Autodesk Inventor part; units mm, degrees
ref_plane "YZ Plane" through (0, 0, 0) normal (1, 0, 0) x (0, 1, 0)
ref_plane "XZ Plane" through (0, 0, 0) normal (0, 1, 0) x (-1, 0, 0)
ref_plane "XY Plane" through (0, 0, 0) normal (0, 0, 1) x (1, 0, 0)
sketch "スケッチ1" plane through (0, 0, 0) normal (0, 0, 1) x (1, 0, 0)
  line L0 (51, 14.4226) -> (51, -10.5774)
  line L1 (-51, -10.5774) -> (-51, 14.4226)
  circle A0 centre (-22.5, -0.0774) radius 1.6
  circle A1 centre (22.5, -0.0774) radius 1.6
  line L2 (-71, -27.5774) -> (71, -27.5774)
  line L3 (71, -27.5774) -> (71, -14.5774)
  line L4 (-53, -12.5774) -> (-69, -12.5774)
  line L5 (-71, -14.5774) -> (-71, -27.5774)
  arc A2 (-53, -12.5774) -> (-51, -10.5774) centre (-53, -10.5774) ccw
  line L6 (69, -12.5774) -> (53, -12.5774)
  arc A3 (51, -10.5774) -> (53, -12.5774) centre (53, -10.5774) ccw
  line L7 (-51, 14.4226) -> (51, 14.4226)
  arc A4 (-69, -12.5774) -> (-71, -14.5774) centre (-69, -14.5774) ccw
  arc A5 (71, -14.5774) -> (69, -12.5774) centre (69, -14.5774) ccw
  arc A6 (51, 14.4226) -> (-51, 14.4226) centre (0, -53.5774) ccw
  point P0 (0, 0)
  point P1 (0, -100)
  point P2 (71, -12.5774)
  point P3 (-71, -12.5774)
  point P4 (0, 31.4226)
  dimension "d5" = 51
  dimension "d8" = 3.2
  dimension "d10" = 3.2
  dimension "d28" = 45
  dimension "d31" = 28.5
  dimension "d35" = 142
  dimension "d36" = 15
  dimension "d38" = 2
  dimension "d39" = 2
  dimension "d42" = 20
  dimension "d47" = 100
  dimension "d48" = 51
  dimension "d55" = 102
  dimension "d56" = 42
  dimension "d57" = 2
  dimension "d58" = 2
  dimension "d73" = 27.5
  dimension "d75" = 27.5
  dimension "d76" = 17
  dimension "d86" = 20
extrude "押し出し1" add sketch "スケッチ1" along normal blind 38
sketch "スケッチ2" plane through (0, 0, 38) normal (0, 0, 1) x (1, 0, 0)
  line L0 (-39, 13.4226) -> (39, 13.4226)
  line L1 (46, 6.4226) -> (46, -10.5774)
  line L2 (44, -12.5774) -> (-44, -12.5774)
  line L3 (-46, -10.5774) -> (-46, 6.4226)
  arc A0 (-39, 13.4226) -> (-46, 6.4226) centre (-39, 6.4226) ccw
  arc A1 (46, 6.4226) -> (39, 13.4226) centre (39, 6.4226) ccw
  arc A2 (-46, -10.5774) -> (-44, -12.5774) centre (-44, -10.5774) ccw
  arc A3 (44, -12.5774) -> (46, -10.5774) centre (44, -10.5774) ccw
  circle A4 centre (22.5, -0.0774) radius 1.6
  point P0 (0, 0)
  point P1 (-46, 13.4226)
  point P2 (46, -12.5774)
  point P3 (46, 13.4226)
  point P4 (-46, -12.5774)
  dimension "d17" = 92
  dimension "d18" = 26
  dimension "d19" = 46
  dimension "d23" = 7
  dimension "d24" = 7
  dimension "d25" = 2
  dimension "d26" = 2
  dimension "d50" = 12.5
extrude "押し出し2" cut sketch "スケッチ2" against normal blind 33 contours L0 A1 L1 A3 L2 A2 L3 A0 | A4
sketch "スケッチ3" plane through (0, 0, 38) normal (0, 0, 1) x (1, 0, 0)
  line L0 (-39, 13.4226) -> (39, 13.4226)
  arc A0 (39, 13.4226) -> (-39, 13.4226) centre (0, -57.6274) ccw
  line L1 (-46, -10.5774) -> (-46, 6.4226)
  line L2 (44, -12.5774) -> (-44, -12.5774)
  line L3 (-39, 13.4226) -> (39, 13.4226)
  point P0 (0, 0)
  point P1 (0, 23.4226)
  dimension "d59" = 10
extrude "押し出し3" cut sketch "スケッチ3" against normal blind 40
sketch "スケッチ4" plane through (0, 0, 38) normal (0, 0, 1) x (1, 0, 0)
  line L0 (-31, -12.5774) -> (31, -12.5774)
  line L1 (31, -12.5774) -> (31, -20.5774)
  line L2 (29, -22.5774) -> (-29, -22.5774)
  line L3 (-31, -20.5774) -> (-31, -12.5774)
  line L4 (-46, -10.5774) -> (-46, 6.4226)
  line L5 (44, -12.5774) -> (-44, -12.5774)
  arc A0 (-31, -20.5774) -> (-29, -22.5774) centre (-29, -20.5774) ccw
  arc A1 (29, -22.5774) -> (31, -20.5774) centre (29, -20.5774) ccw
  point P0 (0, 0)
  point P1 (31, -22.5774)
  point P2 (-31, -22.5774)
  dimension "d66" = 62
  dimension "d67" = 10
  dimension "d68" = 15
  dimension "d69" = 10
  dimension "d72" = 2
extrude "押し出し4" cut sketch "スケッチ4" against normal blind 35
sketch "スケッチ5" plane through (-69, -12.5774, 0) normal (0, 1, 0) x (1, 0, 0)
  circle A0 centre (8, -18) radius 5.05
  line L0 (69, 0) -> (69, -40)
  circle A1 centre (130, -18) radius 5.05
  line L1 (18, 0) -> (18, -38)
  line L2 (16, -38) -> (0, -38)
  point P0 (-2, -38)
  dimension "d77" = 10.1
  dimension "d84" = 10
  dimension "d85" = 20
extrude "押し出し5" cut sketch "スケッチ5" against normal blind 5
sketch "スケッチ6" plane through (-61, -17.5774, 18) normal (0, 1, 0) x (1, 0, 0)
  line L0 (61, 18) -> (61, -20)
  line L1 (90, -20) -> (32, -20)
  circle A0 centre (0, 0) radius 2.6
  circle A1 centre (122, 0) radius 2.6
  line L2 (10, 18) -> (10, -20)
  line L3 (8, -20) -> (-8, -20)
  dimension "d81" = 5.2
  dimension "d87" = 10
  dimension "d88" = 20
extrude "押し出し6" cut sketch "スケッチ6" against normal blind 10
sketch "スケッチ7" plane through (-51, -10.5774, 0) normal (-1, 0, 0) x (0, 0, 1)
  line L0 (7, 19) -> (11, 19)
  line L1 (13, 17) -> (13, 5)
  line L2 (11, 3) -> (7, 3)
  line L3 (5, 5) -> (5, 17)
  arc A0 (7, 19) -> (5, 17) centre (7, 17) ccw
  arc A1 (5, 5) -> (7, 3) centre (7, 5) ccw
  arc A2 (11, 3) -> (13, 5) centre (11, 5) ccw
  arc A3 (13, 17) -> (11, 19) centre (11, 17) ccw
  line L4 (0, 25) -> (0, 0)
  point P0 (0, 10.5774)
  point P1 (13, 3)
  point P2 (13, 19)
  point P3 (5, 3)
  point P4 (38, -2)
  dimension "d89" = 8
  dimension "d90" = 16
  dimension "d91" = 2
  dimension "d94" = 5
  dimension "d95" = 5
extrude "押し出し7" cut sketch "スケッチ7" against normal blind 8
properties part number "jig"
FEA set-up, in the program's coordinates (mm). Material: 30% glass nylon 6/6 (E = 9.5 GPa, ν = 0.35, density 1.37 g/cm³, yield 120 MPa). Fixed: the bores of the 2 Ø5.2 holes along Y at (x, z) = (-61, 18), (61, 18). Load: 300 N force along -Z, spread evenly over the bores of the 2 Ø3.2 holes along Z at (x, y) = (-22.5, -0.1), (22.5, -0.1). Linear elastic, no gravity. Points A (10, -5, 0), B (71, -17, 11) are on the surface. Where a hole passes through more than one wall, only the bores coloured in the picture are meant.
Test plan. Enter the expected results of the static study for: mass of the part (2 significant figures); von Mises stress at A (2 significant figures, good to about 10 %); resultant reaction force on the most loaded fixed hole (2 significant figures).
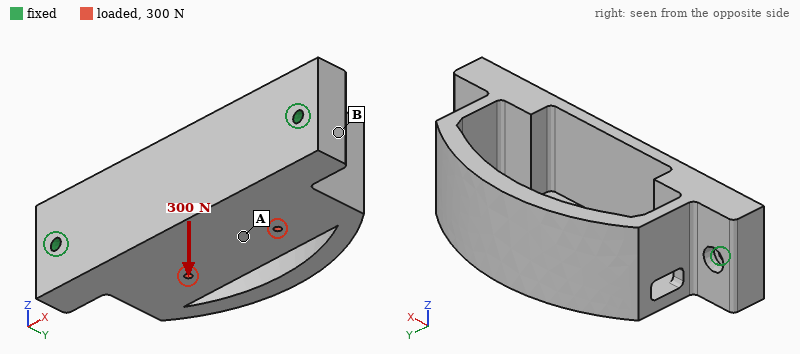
150 g
3.1 MPa
160 N
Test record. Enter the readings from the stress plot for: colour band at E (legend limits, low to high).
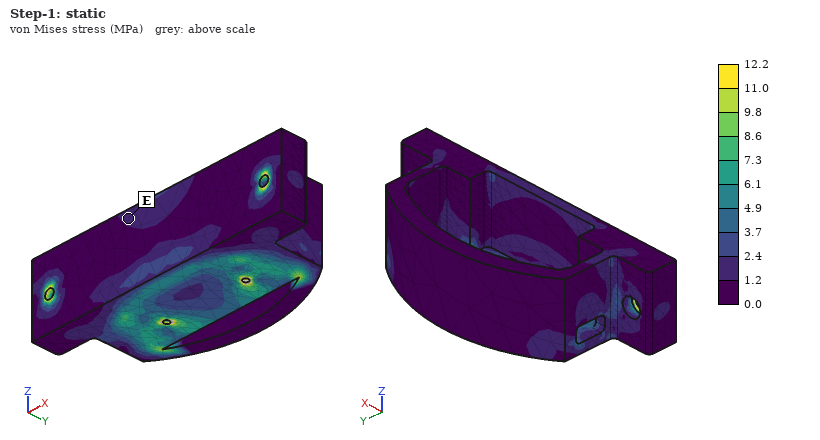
1.2 to 2.4 MPa
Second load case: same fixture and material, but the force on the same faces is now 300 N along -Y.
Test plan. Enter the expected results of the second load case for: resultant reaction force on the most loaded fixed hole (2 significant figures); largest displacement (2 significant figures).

160 N
44 µm
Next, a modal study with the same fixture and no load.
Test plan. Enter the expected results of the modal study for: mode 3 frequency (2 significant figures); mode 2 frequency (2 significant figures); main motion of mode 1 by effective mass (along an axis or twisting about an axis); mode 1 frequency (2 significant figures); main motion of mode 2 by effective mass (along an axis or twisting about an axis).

2300 Hz
1700 Hz
along Z
1000 Hz
along X
